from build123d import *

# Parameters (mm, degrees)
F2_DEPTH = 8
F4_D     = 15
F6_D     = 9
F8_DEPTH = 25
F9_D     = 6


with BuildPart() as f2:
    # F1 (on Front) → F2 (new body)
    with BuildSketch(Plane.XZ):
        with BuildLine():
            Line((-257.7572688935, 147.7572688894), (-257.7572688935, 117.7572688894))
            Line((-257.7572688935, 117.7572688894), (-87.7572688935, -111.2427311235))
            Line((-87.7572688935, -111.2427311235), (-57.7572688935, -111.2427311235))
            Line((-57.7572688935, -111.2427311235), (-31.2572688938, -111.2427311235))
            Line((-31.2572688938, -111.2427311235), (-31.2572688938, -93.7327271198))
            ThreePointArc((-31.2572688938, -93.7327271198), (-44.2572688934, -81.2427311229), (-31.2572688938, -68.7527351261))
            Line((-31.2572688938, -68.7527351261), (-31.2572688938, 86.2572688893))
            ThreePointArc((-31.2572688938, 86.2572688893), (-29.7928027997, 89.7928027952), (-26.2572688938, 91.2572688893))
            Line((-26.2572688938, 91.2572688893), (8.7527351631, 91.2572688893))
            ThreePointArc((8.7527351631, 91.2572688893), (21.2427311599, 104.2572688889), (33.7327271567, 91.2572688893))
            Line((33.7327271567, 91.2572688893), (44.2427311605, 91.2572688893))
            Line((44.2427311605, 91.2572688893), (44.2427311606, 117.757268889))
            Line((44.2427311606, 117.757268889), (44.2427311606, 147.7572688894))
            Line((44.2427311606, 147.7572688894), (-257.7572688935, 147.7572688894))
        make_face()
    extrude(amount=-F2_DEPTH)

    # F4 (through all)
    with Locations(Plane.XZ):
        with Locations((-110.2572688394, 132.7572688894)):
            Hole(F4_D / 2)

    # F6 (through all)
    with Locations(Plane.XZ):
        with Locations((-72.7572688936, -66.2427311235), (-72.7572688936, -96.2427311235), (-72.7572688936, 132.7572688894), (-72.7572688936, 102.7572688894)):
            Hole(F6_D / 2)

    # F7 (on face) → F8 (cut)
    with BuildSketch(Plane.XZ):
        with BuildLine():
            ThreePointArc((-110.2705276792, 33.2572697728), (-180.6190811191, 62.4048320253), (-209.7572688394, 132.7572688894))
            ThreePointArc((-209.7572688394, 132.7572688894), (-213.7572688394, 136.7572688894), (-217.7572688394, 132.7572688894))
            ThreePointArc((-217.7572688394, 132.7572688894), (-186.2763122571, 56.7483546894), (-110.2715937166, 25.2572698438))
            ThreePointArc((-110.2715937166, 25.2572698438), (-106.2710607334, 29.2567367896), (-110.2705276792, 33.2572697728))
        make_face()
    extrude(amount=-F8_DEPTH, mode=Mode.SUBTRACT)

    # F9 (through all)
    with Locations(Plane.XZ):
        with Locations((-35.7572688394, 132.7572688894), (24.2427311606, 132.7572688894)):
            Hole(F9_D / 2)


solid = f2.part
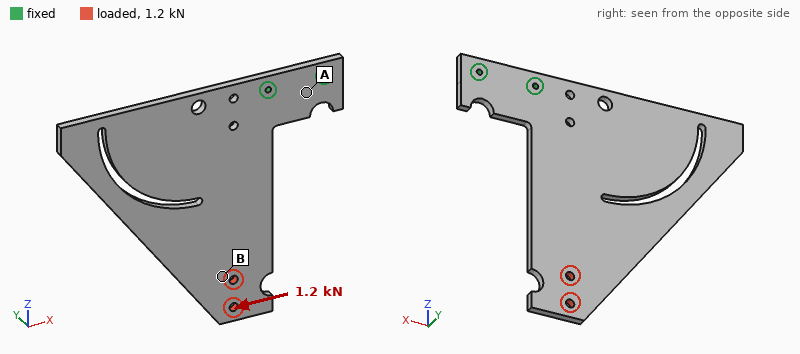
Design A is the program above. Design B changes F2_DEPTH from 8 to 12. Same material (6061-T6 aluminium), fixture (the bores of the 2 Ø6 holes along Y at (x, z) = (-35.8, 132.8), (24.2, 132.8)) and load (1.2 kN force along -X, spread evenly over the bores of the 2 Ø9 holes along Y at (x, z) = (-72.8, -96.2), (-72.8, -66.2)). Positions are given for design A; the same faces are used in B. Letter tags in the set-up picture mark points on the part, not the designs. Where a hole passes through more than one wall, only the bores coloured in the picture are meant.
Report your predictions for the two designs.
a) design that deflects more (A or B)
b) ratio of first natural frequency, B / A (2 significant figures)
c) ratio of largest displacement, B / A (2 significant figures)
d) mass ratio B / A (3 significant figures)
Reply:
A
1.5
0.67
1.50
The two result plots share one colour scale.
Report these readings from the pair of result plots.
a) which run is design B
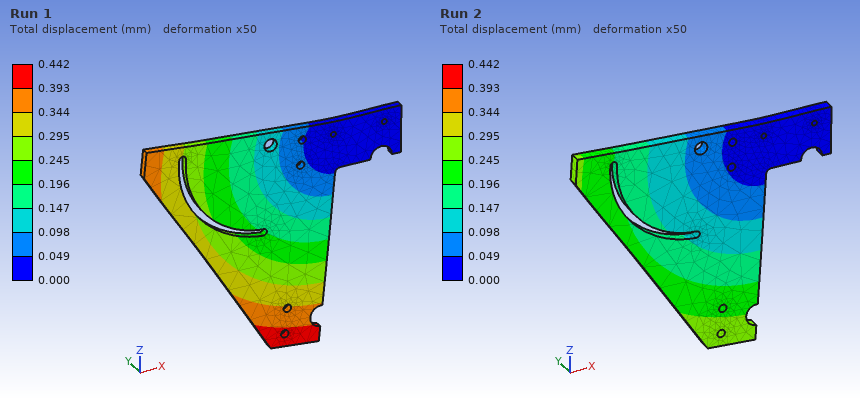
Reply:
Run 2
